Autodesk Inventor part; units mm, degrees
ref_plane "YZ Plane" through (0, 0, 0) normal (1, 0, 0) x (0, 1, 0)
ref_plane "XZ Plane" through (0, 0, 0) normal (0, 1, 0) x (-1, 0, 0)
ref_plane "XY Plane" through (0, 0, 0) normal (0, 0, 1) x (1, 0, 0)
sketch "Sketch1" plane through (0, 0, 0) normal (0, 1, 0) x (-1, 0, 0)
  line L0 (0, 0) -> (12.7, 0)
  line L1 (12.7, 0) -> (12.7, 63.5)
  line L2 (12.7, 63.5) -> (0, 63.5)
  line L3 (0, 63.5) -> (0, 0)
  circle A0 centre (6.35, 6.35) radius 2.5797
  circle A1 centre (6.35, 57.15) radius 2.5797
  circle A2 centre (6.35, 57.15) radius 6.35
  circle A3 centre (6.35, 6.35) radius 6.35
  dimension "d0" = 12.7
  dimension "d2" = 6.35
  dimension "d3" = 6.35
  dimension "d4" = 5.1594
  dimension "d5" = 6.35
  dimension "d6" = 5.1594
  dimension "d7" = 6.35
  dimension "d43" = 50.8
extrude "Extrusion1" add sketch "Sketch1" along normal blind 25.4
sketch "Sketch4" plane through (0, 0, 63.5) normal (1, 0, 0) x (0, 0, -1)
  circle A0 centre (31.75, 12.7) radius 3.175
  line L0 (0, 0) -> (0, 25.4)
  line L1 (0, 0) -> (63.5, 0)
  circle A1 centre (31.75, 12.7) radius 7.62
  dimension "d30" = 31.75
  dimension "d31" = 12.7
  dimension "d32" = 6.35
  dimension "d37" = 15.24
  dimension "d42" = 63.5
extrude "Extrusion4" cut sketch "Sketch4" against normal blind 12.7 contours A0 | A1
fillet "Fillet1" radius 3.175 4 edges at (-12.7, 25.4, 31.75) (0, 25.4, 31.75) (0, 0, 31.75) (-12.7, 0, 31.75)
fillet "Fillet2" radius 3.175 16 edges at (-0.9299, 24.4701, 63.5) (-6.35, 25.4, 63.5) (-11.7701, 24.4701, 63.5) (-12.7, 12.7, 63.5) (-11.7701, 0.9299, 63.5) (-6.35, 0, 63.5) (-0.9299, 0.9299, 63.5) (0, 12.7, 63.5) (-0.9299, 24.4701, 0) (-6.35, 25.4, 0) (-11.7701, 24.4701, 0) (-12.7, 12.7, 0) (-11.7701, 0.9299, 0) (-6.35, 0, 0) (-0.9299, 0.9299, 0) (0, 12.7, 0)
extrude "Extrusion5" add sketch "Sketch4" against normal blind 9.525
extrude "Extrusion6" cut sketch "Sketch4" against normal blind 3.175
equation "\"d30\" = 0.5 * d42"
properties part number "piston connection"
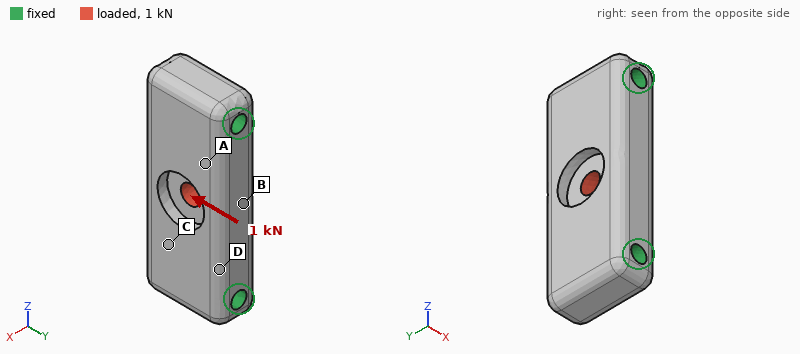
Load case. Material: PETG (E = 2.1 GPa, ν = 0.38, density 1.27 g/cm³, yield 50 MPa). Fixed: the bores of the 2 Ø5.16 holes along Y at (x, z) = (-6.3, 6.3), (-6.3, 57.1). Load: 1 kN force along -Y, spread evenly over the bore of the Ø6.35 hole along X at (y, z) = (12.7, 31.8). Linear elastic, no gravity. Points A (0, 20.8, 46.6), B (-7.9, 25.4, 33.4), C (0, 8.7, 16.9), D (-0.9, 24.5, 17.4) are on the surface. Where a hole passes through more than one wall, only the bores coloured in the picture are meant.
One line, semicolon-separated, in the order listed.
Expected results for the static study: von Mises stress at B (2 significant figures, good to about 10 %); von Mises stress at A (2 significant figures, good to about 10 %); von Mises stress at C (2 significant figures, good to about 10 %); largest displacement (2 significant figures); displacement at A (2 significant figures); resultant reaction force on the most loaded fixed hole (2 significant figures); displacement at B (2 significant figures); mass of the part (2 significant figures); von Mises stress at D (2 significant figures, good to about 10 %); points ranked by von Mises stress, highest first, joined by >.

6.1 MPa; 2.5 MPa; 3.7 MPa; 90 µm; 28 µm; 500 N; 68 µm; 22 g; 1.2 MPa; B > C > A > D
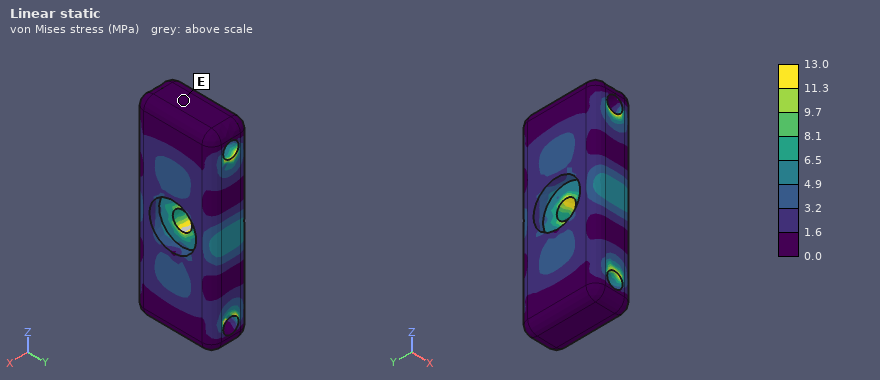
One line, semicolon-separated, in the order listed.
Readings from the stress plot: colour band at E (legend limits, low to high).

0.0 to 1.6 MPa
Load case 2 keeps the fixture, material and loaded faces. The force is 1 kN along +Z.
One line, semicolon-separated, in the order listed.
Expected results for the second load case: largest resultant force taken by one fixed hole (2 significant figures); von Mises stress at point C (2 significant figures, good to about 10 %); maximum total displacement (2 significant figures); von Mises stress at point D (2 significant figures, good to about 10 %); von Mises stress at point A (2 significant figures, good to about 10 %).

500 N; 1.7 MPa; 36 µm; 1.1 MPa; 1.4 MPa
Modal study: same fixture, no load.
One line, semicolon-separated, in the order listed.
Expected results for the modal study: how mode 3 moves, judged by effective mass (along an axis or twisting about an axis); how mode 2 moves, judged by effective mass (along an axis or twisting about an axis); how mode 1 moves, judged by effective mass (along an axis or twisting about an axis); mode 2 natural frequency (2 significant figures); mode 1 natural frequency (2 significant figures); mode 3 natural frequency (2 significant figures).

along Y; twisting about Z; along X; 6600 Hz; 4400 Hz; 7200 Hz
